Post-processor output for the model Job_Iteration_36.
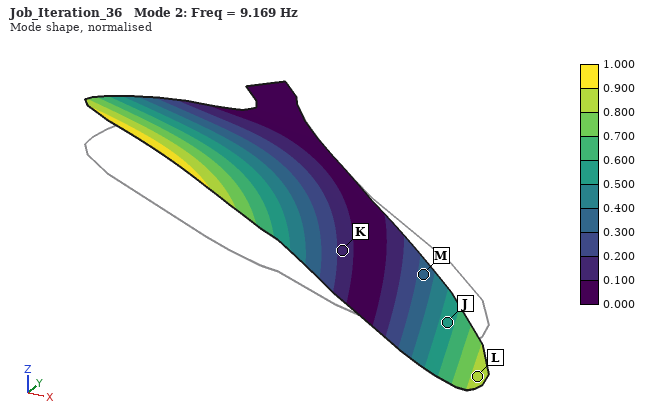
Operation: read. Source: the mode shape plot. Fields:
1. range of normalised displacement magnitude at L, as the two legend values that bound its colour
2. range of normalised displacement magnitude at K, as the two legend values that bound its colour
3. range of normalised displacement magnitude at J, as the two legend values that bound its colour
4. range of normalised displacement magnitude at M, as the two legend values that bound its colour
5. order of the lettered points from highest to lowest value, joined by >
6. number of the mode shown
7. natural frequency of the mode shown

0.800 to 0.900
0.100 to 0.200
0.500 to 0.600
0.300 to 0.400
L > J > M > K
2
9.169 Hz
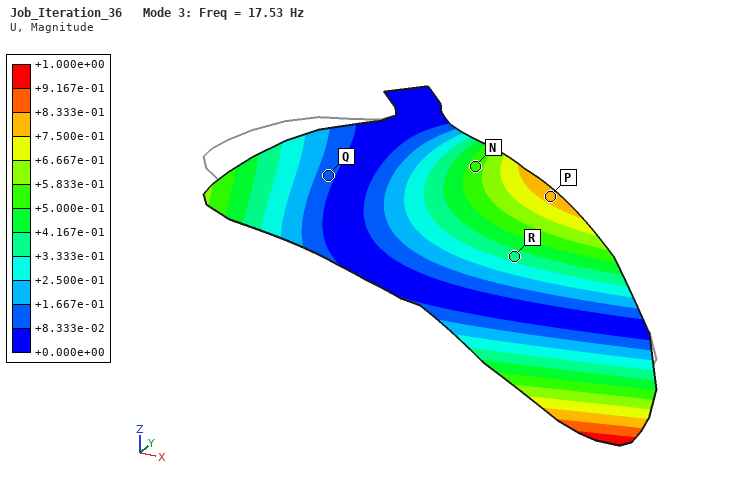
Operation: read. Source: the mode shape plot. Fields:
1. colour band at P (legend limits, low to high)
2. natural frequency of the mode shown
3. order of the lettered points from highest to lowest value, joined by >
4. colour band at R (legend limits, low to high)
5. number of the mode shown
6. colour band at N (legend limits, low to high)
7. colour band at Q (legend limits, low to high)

+7.500e-01 to +8.333e-01
17.53 Hz
P > N > R > Q
+3.333e-01 to +4.167e-01
3
+5.000e-01 to +5.833e-01
+8.333e-02 to +1.667e-01
